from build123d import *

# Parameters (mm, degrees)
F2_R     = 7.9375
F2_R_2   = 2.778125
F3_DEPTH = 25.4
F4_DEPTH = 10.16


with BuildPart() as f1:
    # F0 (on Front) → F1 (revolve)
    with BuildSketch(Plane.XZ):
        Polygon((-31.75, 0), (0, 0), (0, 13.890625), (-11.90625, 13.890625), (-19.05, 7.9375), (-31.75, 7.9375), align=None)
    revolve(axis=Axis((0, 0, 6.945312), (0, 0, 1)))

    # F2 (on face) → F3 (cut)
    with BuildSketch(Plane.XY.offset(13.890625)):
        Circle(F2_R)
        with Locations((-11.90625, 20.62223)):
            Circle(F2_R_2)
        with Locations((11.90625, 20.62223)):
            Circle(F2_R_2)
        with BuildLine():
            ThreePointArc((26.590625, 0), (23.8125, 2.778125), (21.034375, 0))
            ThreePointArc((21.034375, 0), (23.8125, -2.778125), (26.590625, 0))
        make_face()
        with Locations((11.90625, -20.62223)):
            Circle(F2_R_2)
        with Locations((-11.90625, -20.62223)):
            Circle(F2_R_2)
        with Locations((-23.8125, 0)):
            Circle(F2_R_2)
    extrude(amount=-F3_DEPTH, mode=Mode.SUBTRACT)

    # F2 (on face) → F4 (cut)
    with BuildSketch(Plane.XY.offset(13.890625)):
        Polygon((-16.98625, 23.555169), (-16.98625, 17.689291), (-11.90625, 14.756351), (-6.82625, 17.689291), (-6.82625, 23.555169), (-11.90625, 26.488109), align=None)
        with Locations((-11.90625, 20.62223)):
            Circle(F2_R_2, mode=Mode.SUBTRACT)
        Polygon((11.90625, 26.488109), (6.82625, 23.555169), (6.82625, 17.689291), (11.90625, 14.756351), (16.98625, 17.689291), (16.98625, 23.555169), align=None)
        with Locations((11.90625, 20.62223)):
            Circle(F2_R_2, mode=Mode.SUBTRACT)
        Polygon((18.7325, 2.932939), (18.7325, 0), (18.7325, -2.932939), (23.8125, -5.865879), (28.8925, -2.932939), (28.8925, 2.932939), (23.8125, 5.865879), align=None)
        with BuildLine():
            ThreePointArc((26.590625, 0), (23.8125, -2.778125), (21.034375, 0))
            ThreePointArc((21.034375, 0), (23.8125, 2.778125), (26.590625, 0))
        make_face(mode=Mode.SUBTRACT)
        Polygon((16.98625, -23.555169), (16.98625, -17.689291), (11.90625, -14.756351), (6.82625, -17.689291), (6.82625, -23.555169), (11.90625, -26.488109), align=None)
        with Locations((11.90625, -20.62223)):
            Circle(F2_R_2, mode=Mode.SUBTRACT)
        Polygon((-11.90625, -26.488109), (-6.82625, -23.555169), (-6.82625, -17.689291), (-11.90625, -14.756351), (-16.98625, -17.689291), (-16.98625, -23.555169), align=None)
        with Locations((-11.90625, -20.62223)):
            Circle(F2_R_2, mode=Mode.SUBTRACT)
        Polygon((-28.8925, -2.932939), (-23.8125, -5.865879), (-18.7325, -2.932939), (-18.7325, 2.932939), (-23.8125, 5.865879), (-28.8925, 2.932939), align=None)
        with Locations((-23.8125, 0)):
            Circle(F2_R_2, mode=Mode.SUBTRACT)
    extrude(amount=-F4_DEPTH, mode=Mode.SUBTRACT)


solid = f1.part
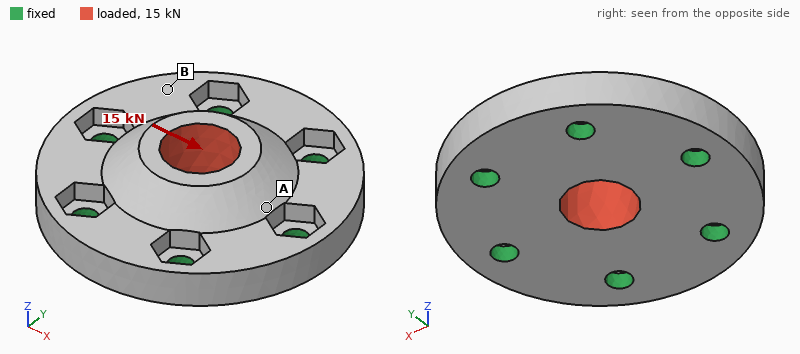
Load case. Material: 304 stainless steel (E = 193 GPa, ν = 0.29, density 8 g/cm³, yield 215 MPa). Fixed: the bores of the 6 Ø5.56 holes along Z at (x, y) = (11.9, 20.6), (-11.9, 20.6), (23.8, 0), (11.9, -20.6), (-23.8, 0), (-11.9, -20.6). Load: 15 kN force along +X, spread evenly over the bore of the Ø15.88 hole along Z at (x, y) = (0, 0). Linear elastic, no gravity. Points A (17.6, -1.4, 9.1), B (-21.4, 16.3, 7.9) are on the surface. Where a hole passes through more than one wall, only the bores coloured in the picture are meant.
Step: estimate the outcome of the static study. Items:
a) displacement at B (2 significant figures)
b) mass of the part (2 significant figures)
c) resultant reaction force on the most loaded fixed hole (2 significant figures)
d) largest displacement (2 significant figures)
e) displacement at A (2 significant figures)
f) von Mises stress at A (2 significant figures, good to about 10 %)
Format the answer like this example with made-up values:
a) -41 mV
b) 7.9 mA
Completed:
a) 2.6 µm
b) 190 g
c) 3.6 kN
d) 5.6 µm
e) 3.6 µm
f) 18 MPa
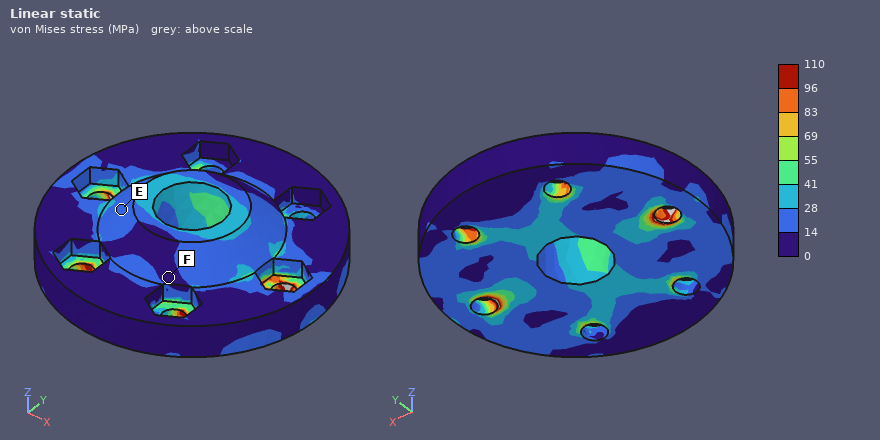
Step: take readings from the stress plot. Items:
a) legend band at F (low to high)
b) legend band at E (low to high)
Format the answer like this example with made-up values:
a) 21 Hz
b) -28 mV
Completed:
a) 0 to 14 MPa
b) 14 to 28 MPa
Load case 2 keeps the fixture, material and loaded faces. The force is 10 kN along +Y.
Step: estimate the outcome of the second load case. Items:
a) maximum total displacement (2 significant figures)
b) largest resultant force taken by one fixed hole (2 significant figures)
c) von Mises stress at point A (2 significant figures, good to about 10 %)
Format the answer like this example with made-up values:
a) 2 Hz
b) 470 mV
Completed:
a) 3.7 µm
b) 2.1 kN
c) 7.4 MPa
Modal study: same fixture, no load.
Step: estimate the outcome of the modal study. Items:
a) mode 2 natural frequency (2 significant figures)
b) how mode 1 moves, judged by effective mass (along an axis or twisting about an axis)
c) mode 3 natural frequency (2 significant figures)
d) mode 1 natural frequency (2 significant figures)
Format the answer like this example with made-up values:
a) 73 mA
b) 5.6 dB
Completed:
a) 28 kHz
b) along Z
c) 28 kHz
d) 24 kHz
